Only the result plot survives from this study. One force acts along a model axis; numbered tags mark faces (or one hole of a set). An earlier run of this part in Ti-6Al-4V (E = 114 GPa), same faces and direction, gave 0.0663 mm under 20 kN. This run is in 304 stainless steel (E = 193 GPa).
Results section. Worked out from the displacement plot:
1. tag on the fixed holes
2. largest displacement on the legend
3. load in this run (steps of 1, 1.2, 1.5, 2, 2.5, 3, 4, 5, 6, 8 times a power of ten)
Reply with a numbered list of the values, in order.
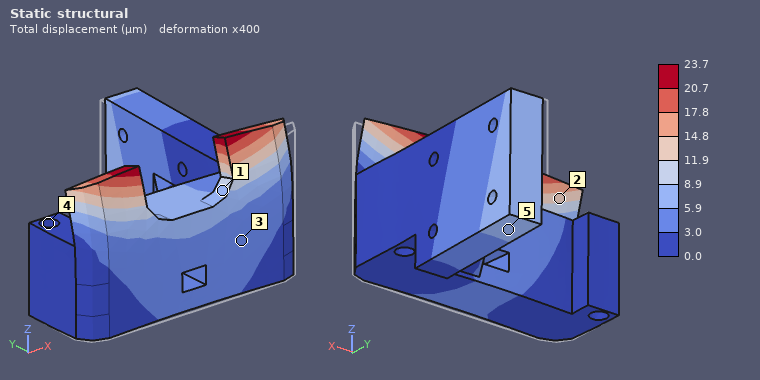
1. 4
2. 23.7 µm
3. 12 kN
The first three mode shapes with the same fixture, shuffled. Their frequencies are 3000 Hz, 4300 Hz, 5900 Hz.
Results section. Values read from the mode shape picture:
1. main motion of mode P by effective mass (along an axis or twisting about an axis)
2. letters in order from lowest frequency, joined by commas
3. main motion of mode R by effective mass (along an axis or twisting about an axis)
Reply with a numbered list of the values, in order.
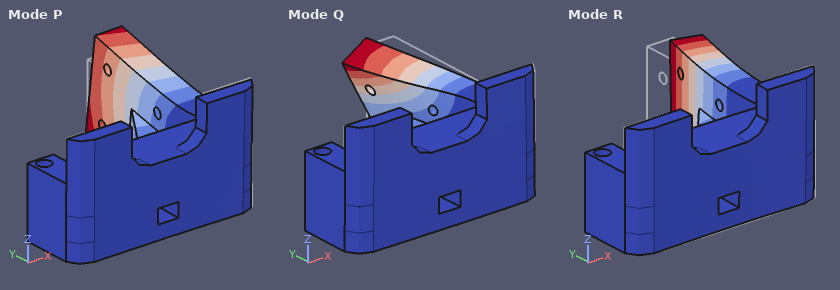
1. along Z
2. R, P, Q
3. along X
